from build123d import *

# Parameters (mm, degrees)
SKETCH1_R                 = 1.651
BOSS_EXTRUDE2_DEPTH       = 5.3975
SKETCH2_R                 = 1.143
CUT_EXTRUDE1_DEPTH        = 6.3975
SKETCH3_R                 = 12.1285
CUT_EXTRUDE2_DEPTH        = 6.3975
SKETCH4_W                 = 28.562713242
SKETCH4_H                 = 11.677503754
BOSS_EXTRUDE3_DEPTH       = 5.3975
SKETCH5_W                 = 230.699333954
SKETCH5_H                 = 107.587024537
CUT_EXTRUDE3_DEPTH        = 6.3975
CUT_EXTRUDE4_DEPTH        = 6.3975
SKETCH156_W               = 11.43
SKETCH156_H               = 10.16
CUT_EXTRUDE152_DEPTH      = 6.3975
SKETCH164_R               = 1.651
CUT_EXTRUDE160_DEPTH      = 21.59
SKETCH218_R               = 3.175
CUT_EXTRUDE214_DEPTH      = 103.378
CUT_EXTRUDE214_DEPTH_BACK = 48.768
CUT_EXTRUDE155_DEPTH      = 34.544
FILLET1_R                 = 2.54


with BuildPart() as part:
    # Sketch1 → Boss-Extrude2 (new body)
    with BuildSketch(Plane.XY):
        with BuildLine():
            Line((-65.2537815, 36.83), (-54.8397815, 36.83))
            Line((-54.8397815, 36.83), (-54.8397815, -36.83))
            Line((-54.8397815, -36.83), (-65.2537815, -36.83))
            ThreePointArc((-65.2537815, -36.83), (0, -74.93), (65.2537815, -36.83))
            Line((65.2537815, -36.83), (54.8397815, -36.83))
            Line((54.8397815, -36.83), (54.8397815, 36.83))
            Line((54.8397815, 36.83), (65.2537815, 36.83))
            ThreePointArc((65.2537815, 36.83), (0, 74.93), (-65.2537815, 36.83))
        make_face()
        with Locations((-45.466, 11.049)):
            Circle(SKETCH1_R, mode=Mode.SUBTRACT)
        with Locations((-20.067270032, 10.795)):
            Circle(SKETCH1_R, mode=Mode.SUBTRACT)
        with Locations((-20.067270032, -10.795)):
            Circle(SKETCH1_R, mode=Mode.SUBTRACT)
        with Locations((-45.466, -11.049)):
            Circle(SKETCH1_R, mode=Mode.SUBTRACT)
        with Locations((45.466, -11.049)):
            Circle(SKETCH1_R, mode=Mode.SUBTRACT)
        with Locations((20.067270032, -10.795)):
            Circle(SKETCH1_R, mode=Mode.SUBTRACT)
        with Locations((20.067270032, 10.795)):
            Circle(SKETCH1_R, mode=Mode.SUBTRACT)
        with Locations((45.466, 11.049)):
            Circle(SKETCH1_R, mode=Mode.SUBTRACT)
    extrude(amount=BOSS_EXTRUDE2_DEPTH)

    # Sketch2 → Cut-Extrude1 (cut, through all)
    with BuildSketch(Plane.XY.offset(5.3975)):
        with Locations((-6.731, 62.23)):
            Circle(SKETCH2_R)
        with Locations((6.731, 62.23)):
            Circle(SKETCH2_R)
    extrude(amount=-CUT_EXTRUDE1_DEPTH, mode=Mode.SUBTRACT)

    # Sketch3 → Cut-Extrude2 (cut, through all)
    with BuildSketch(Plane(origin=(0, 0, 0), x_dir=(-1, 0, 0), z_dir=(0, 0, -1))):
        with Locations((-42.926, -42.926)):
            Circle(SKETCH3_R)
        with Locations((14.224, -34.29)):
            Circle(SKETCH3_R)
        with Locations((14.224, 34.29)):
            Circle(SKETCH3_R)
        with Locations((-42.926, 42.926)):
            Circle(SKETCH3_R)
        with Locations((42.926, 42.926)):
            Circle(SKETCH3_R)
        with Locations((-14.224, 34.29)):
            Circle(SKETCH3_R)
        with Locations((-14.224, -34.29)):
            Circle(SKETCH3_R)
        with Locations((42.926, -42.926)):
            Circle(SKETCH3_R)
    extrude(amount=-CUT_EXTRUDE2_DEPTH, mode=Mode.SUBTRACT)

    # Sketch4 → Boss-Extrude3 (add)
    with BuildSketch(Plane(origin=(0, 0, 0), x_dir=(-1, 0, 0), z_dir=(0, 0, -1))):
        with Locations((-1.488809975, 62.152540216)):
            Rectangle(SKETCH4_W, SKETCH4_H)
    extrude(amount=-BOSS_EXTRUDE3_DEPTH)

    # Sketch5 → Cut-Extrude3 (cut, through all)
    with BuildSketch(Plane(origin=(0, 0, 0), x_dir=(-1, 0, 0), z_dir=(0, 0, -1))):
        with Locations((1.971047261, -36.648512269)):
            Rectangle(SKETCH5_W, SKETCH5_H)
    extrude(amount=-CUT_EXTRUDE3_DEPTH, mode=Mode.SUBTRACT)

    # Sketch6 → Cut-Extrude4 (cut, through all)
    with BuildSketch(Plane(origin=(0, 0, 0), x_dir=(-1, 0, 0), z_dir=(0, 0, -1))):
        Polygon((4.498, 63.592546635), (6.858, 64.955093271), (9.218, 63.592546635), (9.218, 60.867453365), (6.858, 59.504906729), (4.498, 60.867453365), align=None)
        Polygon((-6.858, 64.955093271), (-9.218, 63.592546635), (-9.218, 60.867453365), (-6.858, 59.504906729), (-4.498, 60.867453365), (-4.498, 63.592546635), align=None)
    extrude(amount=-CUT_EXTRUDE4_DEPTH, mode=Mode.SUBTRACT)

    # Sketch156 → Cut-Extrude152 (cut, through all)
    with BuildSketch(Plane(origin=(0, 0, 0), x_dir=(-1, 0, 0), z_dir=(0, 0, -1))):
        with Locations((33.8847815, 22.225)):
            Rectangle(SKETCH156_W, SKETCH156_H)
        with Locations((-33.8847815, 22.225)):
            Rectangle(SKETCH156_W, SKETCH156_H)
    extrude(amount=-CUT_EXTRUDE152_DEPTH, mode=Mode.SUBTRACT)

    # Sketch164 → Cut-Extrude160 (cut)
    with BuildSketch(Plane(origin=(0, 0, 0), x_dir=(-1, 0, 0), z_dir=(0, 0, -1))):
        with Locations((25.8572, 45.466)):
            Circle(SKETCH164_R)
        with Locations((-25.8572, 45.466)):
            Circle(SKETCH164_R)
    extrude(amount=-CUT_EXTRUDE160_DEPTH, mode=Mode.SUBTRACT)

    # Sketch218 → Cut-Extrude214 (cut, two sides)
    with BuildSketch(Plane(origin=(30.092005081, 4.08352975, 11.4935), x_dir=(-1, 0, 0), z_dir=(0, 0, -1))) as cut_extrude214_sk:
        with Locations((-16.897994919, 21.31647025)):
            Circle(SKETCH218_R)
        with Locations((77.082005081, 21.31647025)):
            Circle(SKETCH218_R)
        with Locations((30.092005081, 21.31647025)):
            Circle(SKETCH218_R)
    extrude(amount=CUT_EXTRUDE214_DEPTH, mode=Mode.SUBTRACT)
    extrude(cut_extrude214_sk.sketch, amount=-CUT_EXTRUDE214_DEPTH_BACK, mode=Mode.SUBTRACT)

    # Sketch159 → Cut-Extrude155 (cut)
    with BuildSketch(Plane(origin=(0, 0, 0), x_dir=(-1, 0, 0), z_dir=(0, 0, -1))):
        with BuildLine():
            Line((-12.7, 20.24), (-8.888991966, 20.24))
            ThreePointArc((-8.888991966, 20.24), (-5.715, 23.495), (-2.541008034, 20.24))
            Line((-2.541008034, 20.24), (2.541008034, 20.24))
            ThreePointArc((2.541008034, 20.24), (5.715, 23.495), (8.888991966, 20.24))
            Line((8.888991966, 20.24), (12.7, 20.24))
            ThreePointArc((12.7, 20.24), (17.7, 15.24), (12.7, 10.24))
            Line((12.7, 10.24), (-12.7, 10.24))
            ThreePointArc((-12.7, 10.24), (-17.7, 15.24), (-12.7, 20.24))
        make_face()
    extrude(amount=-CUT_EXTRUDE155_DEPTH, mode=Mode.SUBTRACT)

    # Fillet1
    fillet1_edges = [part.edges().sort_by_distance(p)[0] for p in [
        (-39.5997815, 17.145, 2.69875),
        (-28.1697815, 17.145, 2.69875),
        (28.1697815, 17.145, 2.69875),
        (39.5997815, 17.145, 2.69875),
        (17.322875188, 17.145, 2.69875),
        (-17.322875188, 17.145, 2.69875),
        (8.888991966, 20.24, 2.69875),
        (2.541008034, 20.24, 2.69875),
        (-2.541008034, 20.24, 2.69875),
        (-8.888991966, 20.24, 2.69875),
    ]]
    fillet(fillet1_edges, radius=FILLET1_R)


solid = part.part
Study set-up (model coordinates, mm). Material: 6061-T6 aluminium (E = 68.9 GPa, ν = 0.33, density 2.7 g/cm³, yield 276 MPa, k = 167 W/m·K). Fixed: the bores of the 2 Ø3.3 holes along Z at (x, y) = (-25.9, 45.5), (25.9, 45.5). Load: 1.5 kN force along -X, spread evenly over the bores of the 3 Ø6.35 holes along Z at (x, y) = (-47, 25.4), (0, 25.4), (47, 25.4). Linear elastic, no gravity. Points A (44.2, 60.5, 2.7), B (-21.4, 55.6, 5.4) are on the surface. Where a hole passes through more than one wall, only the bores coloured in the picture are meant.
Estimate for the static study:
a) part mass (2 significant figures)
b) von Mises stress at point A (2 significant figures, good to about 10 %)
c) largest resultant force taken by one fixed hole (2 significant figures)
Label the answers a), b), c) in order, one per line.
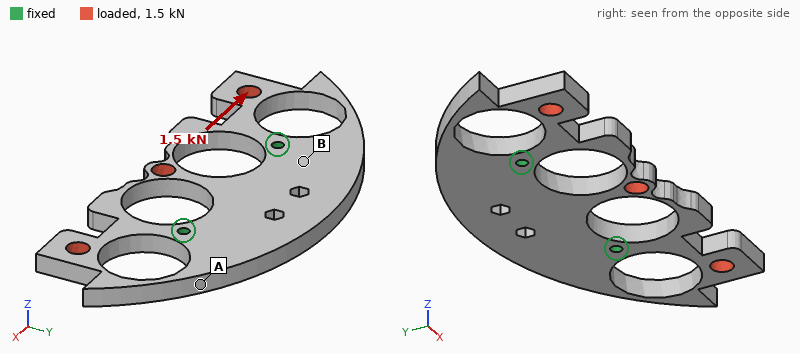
a) 48 g
b) 44 MPa
c) 880 N
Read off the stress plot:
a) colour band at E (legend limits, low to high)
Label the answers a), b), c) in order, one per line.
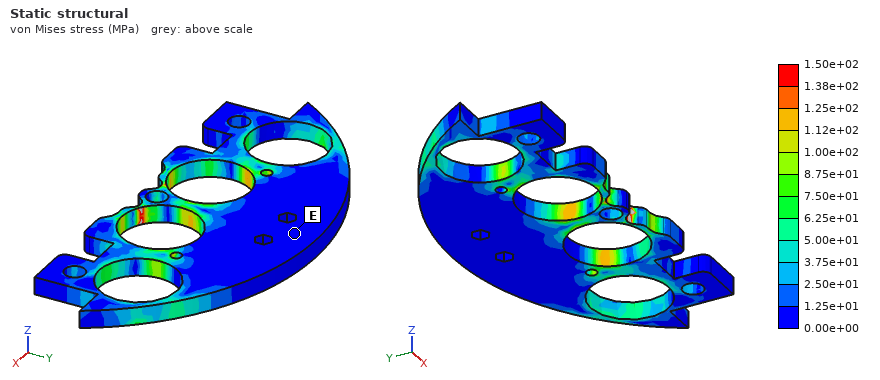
a) 0.00e+00 to 1.25e+01 MPa
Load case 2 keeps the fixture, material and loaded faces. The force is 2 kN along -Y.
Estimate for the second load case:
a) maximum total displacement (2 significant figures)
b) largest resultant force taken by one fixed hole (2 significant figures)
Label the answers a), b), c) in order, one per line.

a) 0.11 mm
b) 1.0 kN
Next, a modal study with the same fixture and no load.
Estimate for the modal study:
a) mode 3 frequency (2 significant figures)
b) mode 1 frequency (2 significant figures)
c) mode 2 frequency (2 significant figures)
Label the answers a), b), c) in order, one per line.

a) 3500 Hz
b) 2200 Hz
c) 2300 Hz
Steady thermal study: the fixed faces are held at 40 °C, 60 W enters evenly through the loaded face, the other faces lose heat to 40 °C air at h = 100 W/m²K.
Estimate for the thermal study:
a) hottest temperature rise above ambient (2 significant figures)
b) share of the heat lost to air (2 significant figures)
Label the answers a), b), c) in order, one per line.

a) 66 K
b) 39 %
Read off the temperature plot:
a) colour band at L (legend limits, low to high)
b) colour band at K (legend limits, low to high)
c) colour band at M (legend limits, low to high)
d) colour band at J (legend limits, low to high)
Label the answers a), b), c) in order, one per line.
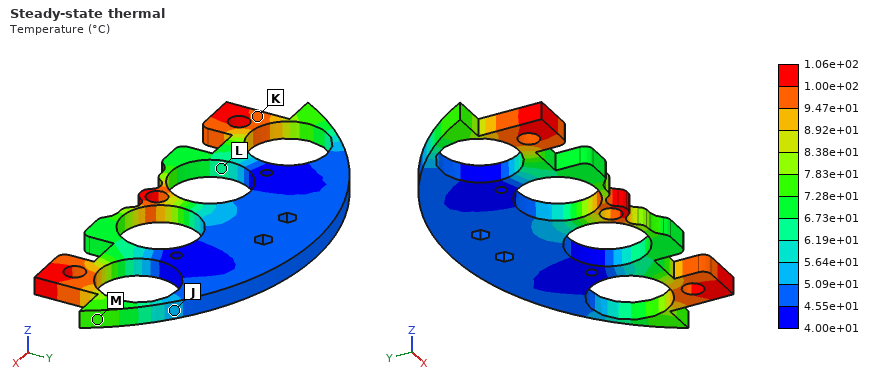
a) 6.19e+01 to 6.73e+01 °C
b) 9.47e+01 to 1.00e+02 °C
c) 7.28e+01 to 7.83e+01 °C
d) 5.09e+01 to 5.64e+01 °C
